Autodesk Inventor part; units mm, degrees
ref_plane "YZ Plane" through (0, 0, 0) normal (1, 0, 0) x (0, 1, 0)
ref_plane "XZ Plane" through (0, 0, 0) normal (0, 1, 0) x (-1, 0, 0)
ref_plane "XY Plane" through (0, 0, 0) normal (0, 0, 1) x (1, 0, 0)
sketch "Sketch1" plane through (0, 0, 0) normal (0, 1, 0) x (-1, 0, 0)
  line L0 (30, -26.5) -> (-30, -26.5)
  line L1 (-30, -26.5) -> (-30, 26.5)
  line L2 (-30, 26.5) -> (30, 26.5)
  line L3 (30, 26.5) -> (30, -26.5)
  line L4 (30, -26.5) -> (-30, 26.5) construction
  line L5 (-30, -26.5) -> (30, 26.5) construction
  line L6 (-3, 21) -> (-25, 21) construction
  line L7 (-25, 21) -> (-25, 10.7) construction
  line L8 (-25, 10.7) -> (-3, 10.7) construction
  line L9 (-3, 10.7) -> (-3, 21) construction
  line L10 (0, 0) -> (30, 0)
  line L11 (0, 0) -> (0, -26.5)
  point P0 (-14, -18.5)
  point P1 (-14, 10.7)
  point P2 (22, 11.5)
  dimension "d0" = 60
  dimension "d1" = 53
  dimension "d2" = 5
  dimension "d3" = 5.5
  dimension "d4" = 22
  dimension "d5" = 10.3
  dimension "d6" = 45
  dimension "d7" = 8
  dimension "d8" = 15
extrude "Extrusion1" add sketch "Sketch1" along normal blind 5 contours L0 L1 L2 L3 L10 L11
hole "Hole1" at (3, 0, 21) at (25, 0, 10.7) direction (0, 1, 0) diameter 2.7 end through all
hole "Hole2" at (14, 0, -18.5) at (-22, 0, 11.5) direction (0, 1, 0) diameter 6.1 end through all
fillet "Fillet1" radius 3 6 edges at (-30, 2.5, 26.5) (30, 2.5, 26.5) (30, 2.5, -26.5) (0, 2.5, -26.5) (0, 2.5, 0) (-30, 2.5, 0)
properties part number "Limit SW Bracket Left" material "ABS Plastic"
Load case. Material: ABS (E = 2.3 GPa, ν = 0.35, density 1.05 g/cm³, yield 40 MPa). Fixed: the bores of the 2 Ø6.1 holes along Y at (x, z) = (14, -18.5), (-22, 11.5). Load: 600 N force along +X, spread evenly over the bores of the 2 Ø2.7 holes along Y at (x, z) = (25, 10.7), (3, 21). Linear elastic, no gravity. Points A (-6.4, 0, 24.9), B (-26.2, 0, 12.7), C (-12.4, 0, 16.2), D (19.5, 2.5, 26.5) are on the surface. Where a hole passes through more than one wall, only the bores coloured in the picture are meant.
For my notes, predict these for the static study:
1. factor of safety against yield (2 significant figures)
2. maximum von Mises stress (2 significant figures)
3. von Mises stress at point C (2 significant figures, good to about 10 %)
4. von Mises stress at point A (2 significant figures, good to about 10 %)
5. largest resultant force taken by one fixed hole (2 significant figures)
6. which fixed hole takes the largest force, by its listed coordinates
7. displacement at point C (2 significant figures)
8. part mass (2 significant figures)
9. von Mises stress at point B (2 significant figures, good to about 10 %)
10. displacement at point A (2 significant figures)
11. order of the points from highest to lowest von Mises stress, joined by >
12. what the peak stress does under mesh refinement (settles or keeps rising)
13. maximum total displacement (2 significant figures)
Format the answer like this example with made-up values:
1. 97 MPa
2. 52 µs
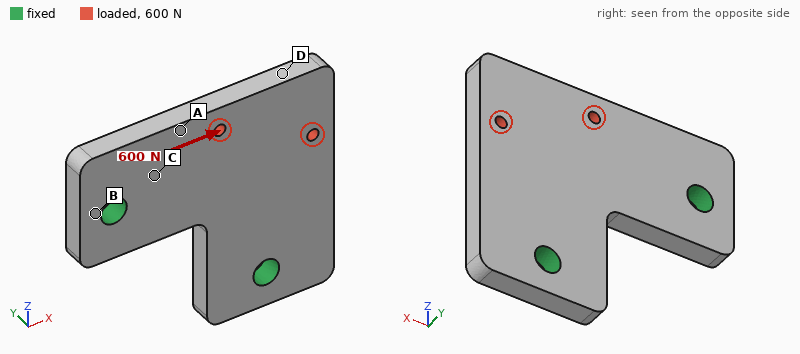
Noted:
1. 2.5
2. 16 MPa
3. 6.4 MPa
4. 4.7 MPa
5. 540 N
6. (-22, 11.5)
7. 0.029 mm
8. 12 g
9. 2.5 MPa
10. 0.054 mm
11. C > A > B > D
12. settles
13. 0.10 mm
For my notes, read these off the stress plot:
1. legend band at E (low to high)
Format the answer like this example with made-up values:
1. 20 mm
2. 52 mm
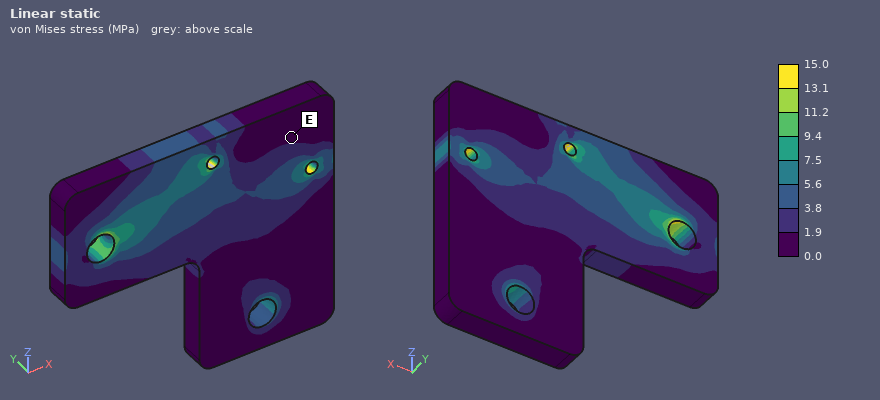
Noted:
1. 0.0 to 1.9 MPa
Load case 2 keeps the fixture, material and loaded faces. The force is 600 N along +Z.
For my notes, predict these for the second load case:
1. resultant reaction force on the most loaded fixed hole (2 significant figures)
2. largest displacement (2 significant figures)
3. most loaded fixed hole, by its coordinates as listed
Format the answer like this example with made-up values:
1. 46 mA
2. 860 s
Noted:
1. 530 N
2. 85 µm
3. (14, -18.5)
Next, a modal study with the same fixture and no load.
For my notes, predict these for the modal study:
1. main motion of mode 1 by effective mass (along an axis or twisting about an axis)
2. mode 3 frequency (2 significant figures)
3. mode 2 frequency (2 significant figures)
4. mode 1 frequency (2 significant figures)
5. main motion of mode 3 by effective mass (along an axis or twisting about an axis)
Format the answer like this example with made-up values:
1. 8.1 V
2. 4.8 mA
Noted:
1. along Y
2. 3700 Hz
3. 2800 Hz
4. 940 Hz
5. along Y
